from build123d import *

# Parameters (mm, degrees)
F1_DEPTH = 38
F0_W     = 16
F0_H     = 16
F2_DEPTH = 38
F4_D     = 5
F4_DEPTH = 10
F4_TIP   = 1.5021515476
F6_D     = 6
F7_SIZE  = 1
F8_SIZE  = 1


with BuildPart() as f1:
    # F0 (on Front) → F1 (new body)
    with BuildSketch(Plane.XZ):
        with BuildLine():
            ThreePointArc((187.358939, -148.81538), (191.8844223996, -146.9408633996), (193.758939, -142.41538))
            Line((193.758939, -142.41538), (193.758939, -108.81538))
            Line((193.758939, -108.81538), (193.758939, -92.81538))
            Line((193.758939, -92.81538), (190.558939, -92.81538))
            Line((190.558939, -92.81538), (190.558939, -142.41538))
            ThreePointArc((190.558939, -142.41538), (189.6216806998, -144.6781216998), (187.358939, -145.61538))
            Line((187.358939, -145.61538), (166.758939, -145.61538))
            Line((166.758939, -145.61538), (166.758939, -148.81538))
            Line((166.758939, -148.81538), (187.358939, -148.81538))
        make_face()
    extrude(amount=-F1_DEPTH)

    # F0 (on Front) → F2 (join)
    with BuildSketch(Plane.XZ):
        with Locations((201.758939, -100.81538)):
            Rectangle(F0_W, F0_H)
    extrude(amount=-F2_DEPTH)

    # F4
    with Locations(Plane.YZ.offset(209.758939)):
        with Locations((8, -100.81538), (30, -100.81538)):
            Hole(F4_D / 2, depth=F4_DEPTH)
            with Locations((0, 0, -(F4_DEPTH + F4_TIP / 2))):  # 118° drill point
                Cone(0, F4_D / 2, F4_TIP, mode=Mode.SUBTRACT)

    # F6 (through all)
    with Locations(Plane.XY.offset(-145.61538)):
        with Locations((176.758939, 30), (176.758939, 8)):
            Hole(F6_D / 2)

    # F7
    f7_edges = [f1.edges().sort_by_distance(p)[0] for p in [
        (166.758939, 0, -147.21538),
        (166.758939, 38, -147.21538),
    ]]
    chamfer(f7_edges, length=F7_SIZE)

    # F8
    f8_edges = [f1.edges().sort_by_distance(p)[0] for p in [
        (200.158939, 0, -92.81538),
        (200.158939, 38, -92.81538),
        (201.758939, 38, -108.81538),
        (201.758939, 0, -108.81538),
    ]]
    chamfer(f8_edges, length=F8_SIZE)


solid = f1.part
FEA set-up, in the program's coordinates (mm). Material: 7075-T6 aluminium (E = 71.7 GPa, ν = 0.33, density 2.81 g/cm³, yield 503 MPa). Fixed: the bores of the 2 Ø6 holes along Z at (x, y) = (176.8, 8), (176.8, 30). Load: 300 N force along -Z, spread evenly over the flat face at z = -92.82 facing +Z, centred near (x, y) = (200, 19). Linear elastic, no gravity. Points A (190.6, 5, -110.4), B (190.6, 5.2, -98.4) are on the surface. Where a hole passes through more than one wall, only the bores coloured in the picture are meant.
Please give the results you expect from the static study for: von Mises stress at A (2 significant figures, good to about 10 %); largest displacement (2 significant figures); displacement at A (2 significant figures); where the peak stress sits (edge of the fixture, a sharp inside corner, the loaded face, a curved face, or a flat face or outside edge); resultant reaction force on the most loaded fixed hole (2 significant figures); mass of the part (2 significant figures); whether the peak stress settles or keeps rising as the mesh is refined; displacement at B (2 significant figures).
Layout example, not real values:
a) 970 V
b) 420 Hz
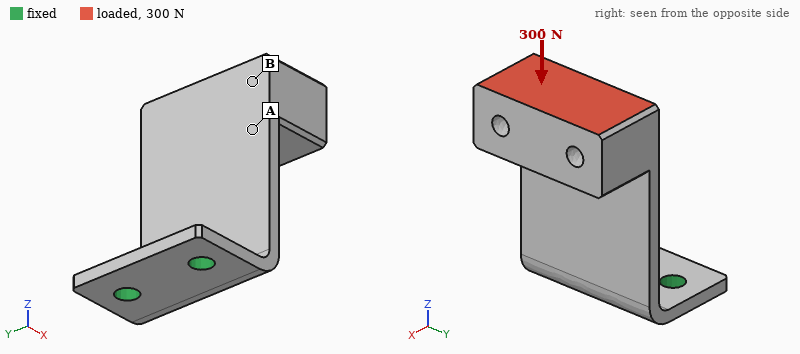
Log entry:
a) 28 MPa
b) 0.91 mm
c) 0.47 mm
d) edge of the fixture
e) 150 N
f) 52 g
g) keeps rising
h) 0.70 mm
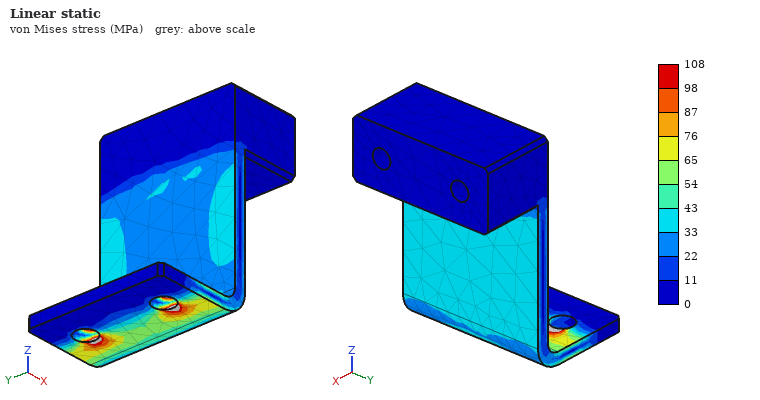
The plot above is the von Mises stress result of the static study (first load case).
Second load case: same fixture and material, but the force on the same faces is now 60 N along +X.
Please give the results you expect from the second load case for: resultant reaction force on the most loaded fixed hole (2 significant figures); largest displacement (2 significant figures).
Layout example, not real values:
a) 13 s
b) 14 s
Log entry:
a) 40 N
b) 0.73 mm
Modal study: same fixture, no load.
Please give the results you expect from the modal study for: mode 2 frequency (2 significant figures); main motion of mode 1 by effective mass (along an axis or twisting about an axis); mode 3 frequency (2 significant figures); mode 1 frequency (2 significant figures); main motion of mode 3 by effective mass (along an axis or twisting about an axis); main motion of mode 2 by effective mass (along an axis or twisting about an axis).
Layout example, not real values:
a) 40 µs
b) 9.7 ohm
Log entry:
a) 950 Hz
b) along X
c) 1300 Hz
d) 300 Hz
e) twisting about Z
f) along Y
